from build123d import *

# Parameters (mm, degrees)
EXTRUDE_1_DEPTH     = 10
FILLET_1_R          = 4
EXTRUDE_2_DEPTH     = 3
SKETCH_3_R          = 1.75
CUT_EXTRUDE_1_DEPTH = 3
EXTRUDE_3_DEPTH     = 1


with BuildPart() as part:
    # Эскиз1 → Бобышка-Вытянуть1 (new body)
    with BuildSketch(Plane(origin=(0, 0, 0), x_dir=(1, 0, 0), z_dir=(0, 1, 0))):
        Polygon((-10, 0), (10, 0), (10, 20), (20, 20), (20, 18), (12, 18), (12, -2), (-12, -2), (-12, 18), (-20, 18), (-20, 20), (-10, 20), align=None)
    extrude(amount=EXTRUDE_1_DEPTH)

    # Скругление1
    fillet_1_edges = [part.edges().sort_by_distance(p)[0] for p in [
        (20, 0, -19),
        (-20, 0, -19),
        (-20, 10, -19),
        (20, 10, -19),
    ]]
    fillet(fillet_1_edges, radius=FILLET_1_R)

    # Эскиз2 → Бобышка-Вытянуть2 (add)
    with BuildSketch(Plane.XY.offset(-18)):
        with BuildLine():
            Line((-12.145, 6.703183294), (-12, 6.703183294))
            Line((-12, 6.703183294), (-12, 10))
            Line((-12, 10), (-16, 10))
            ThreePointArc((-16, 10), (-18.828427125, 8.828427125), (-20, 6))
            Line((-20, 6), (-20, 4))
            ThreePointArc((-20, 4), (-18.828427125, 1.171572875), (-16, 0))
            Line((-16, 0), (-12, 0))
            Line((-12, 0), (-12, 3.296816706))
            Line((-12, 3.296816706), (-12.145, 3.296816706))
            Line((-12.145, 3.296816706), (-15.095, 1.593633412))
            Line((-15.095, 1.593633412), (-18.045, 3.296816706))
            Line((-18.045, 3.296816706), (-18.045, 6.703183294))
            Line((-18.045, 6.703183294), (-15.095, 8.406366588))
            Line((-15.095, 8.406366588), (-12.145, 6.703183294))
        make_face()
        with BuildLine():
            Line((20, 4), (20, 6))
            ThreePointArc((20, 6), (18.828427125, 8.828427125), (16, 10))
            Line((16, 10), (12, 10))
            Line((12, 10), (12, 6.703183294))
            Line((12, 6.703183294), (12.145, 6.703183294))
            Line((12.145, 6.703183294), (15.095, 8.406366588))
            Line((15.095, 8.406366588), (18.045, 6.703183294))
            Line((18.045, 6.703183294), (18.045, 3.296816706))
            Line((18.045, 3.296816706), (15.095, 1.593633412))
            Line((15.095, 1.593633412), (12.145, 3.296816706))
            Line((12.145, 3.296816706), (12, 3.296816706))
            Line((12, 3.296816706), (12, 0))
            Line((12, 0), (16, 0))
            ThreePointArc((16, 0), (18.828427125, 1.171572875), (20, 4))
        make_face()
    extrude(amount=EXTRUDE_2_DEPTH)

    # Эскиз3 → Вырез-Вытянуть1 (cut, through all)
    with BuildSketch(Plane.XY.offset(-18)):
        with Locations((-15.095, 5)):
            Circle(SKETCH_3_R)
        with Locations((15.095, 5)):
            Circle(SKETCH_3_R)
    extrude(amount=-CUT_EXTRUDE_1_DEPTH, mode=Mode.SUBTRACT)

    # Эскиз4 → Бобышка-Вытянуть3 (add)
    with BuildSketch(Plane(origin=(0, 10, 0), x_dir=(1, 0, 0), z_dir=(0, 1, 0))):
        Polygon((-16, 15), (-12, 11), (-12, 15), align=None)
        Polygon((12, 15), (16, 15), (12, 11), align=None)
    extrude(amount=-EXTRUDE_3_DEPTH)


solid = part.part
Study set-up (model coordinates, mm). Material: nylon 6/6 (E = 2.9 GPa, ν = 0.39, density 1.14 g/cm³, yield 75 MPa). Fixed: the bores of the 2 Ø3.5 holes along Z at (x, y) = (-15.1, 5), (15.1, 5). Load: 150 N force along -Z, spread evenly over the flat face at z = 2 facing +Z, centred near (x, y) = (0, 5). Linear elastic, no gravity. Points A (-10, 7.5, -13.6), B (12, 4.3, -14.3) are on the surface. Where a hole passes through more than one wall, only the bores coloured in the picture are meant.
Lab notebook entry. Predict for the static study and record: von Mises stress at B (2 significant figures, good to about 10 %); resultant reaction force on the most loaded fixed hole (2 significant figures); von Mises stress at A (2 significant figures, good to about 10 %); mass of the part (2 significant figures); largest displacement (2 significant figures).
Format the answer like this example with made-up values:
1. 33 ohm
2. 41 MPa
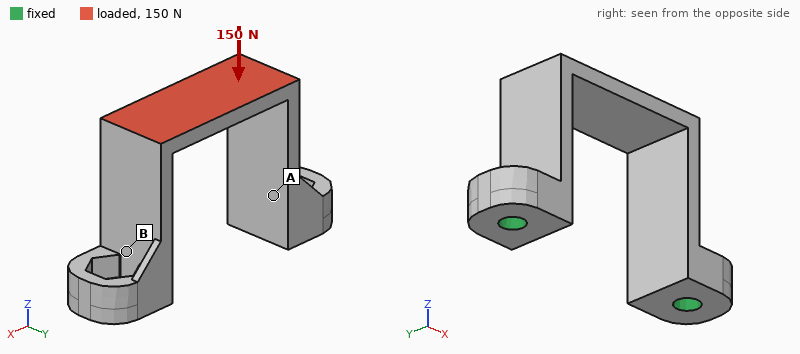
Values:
1. 10.0 MPa
2. 77 N
3. 4.1 MPa
4. 2.1 g
5. 0.42 mm
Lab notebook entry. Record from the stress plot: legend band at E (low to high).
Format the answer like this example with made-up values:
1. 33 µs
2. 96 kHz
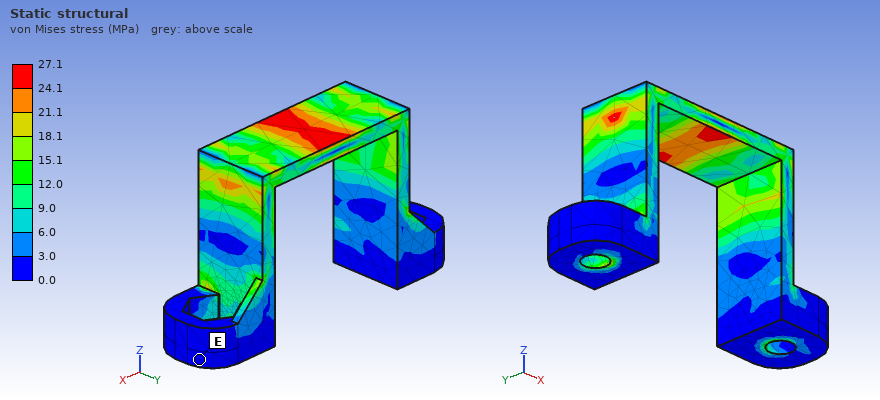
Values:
1. 0.0 to 3.0 MPa
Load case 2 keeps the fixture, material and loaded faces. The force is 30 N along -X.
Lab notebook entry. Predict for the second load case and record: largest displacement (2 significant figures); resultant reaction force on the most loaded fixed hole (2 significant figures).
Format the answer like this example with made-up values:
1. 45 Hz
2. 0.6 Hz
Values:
1. 0.46 mm
2. 19 N
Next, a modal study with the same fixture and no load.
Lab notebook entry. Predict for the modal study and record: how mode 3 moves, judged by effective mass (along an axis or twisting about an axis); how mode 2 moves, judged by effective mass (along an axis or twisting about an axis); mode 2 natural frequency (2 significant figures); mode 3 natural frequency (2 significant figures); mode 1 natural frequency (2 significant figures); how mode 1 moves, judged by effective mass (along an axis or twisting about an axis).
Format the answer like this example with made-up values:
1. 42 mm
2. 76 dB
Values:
1. twisting about Z
2. along Y
3. 1900 Hz
4. 2600 Hz
5. 1500 Hz
6. along X
